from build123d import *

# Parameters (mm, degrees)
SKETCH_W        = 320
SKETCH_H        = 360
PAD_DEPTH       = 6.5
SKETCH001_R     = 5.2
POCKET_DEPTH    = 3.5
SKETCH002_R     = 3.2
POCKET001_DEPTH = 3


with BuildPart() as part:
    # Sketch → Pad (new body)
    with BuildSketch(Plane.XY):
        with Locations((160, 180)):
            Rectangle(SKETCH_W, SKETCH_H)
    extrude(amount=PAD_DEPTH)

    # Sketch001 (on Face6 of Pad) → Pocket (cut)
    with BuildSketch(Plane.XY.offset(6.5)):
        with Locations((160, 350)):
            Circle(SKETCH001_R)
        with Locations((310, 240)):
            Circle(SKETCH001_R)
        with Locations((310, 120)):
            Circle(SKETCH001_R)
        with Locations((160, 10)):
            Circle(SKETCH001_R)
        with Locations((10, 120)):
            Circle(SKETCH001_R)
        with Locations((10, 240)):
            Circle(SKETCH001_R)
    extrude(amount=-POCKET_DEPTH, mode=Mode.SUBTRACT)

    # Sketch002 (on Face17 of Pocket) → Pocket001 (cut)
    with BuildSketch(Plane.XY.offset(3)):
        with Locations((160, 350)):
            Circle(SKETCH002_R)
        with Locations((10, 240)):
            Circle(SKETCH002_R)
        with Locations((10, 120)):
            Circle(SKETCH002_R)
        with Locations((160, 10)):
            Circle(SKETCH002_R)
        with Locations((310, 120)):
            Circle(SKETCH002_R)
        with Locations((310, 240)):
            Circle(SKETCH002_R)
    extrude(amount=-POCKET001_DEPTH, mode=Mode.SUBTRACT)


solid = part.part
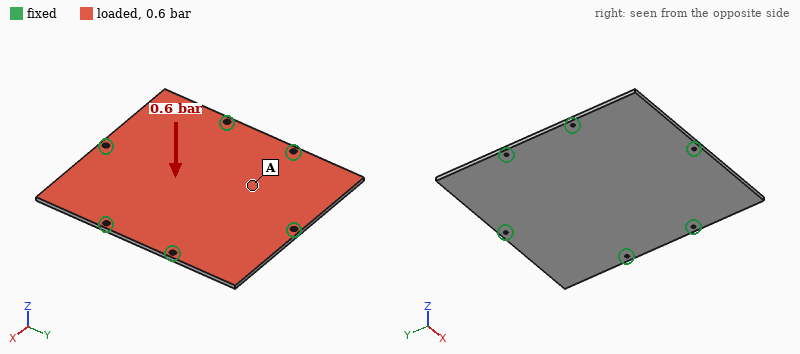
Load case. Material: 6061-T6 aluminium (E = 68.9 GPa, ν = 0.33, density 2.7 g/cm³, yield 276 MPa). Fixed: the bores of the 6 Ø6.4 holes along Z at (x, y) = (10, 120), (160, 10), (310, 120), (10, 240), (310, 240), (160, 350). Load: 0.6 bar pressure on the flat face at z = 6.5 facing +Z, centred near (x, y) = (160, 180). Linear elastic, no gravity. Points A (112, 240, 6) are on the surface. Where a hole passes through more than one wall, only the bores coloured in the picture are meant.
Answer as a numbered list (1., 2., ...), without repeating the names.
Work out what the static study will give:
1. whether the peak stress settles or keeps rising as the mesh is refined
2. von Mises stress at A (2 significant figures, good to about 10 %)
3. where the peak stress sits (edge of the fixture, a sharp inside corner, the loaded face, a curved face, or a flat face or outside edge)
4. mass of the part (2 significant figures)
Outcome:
1. keeps rising
2. 23 MPa
3. edge of the fixture
4. 2.0 kg
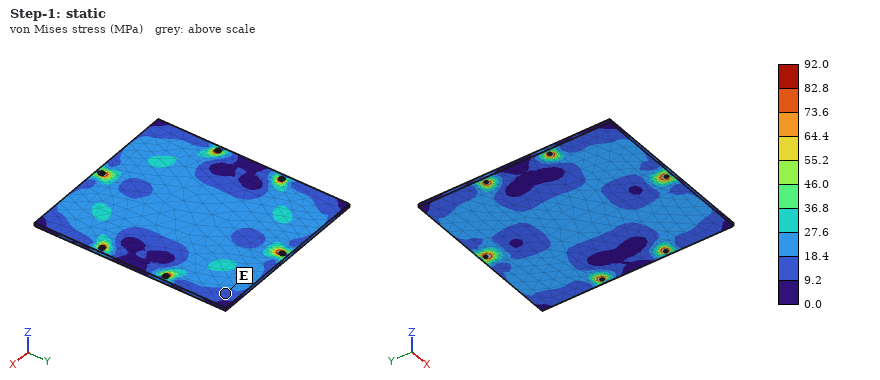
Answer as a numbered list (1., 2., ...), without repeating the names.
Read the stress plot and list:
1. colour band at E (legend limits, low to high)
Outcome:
1. 9.2 to 18.4 MPa
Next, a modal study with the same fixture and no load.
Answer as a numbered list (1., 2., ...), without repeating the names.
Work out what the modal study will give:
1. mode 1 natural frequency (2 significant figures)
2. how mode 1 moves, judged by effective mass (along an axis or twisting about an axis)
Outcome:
1. 390 Hz
2. along Z
